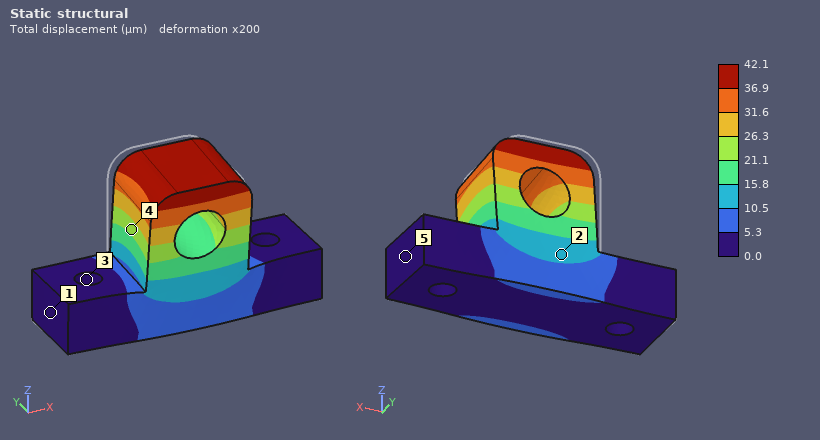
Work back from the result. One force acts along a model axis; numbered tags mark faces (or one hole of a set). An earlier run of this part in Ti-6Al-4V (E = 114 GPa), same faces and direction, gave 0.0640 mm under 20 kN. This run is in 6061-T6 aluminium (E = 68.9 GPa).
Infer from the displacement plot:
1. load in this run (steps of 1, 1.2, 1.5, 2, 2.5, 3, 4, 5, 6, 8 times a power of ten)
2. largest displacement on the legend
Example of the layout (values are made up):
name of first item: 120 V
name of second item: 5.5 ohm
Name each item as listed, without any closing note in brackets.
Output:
load in this run: 8 kN
largest displacement on the legend: 42.1 µm
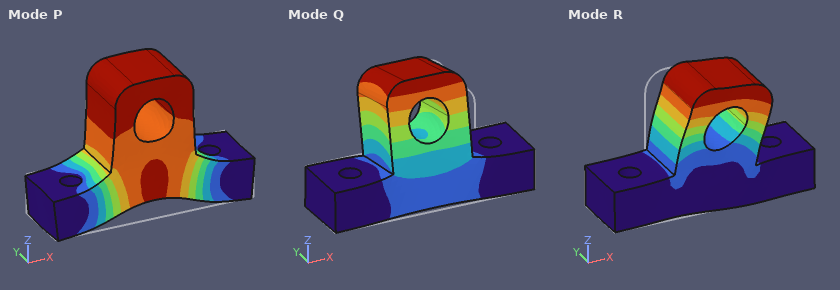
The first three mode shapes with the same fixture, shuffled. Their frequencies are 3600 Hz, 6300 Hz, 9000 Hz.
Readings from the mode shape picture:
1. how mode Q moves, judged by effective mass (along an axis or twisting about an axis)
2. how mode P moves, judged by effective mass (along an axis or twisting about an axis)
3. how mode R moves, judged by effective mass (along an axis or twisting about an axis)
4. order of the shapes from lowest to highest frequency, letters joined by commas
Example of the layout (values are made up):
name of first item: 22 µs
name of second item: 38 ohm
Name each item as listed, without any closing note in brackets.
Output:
how mode Q moves, judged by effective mass: along Y
how mode P moves, judged by effective mass: along Z
how mode R moves, judged by effective mass: along X
order of the shapes from lowest to highest frequency, letters joined by commas: Q, R, P
